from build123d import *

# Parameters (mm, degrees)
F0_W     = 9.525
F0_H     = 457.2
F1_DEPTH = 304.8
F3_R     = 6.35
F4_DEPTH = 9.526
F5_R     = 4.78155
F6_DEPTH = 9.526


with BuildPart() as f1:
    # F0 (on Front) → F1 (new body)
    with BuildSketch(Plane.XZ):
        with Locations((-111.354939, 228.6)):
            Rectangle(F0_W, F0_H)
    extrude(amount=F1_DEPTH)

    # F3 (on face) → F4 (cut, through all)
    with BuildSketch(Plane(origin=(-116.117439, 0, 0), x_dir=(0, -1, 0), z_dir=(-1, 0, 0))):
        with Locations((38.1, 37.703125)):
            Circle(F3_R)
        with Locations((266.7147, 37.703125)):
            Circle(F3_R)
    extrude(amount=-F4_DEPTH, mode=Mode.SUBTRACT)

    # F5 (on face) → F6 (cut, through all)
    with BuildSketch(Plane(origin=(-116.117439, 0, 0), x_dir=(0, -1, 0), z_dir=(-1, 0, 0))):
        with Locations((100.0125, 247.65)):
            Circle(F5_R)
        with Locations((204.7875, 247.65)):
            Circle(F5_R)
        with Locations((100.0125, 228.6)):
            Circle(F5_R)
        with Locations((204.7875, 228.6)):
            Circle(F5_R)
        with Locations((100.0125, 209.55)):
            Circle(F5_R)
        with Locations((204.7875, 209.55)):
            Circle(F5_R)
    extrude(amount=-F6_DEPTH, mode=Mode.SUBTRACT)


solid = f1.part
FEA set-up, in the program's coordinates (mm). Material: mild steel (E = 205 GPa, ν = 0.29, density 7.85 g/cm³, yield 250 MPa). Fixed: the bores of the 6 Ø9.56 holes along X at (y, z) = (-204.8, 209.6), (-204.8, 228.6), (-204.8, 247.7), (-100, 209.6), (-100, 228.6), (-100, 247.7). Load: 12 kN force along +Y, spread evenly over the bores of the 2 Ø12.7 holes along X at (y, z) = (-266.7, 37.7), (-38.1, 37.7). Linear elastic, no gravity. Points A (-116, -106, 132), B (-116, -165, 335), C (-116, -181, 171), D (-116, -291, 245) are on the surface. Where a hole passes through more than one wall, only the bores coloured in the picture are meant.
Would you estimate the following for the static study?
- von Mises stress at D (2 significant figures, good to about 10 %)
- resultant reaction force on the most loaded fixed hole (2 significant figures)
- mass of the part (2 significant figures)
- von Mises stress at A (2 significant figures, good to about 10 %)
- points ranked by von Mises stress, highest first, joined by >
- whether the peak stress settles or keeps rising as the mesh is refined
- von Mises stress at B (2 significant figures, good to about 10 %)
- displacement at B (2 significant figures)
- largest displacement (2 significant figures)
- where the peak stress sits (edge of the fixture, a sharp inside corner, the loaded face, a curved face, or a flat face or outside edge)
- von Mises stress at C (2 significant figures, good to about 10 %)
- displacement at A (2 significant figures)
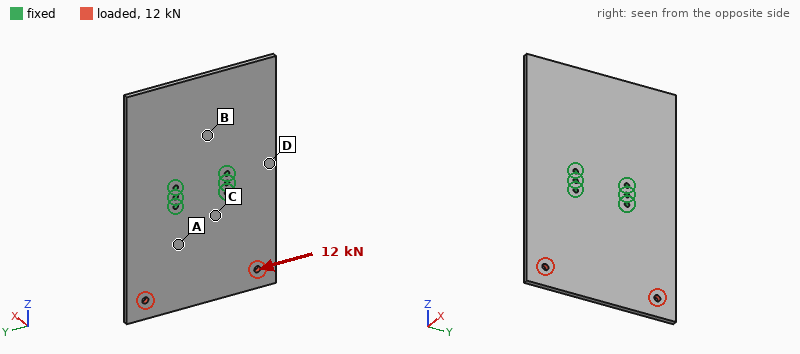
6.6 MPa
11 kN
10 kg
12 MPa
C > A > D > B
keeps rising
3.2 MPa
7.4 µm
43 µm
edge of the fixture
18 MPa
15 µm
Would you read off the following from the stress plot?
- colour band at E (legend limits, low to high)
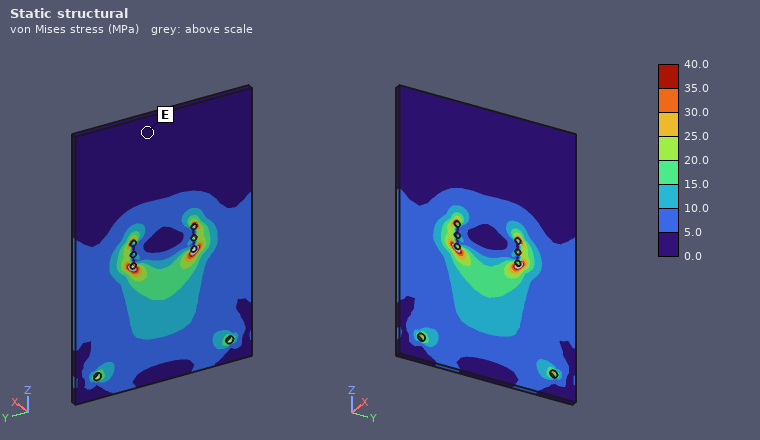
0.0 to 5.0 MPa
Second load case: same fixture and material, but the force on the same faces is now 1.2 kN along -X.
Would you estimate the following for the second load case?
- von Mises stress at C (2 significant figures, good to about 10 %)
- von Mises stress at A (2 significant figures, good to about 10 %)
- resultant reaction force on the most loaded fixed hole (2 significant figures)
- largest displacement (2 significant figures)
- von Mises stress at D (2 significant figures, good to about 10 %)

35 MPa
22 MPa
2.4 kN
0.71 mm
12 MPa
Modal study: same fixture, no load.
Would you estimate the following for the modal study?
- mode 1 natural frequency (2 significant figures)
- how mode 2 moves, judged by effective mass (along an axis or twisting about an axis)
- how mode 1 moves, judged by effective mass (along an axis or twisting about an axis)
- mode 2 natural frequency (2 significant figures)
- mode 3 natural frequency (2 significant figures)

160 Hz
along X
twisting about Y
170 Hz
280 Hz
